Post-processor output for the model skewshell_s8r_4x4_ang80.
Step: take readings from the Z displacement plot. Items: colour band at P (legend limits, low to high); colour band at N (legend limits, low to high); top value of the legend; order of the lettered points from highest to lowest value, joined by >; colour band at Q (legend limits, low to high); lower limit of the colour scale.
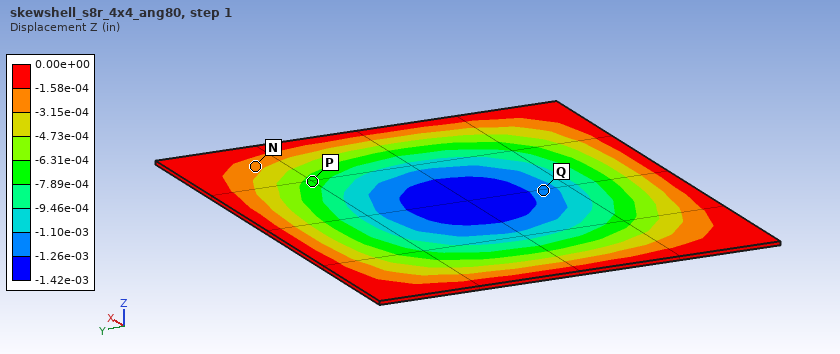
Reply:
-7.89e-04 to -6.31e-04 in
-3.15e-04 to -1.58e-04 in
0.00e+00 in
N > P > Q
-1.26e-03 to -1.10e-03 in
-1.42e-03 in
